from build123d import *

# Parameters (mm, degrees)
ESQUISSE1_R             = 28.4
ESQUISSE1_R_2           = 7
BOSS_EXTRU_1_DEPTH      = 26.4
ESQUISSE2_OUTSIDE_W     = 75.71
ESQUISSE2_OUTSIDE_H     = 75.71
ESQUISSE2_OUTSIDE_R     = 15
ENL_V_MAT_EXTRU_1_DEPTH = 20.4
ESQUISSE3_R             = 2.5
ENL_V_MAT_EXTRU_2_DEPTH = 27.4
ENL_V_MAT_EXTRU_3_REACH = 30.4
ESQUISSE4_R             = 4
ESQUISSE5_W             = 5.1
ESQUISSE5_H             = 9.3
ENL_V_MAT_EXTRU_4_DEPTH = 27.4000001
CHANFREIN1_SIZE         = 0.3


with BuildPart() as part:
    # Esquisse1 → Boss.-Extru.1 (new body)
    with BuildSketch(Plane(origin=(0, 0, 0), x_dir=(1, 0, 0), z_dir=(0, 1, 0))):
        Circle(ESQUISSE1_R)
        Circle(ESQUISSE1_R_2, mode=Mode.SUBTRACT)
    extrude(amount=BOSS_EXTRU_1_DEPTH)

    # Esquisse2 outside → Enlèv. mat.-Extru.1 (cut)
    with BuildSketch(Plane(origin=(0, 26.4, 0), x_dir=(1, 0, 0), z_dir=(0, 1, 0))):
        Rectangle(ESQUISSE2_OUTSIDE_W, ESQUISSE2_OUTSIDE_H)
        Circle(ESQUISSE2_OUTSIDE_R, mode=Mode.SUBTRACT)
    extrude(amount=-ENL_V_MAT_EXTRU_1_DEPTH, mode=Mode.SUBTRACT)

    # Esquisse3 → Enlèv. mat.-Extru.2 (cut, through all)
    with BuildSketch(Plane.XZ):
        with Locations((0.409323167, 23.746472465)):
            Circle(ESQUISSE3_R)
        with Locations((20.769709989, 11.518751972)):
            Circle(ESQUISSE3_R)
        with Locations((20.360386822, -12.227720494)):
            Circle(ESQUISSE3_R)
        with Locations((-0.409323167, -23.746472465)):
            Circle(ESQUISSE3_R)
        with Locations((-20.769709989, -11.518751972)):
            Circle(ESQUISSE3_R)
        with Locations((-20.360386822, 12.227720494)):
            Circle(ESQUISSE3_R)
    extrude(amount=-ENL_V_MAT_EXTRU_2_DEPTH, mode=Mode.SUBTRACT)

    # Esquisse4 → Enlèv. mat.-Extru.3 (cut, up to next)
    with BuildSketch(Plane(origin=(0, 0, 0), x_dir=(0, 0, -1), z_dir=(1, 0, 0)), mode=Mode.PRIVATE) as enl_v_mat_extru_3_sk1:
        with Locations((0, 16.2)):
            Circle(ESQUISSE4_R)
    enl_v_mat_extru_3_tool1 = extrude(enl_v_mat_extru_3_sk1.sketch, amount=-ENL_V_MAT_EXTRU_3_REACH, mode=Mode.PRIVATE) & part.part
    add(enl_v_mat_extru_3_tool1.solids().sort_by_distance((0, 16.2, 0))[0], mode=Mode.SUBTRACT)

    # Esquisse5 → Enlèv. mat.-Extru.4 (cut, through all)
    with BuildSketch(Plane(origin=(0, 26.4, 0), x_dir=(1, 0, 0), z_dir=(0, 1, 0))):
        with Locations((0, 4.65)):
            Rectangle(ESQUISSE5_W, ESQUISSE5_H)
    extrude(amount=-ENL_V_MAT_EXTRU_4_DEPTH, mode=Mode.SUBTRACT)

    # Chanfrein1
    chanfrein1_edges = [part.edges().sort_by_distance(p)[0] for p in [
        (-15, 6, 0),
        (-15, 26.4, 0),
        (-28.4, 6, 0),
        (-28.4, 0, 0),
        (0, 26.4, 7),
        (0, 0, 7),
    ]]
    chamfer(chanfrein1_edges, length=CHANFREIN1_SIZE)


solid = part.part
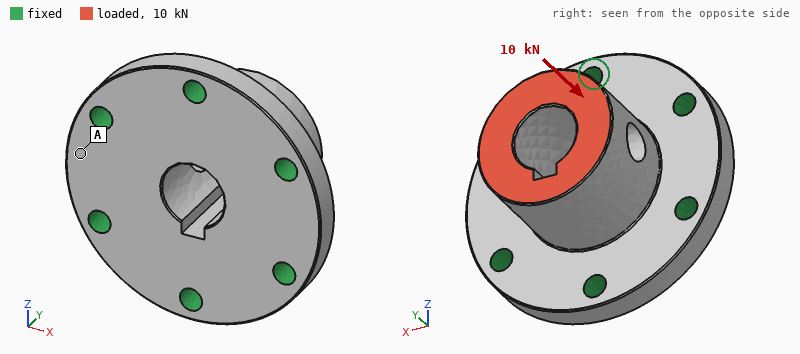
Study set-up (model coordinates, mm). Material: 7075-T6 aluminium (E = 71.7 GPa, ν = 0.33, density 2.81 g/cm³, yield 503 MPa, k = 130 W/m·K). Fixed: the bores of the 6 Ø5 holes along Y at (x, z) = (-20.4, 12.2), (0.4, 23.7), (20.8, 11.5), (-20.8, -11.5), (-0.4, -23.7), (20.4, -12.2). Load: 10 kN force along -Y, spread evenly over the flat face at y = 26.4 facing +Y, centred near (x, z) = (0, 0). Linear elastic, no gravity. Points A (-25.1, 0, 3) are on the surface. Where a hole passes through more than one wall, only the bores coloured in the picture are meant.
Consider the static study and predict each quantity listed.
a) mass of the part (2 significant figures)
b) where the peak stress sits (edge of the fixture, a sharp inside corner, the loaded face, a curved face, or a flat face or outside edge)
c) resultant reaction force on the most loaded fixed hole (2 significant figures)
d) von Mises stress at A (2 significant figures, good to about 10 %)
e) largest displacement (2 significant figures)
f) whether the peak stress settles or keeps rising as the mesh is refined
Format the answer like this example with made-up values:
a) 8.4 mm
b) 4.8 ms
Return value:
a) 68 g
b) edge of the fixture
c) 1.9 kN
d) 15 MPa
e) 26 µm
f) keeps rising
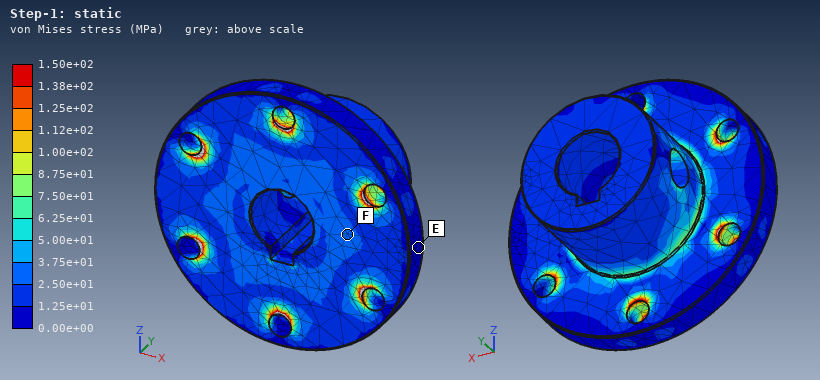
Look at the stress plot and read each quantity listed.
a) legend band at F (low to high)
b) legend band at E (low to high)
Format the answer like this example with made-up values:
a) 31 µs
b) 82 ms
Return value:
a) 2.50e+01 to 3.75e+01 MPa
b) 0.00e+00 to 1.25e+01 MPa
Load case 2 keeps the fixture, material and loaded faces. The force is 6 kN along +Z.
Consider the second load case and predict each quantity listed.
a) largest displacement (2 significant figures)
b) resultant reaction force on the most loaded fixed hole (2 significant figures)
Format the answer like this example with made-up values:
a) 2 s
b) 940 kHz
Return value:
a) 60 µm
b) 2.8 kN
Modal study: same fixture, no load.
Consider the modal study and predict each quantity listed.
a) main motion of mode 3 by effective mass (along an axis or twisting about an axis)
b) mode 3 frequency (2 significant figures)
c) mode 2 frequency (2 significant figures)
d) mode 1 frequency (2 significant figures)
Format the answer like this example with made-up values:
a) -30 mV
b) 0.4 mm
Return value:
a) along Y
b) 18 kHz
c) 15 kHz
d) 15 kHz
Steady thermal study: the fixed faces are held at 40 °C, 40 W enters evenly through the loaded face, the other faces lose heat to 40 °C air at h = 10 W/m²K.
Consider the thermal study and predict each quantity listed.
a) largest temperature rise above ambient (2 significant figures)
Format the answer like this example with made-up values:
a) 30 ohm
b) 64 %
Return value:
a) 20 K
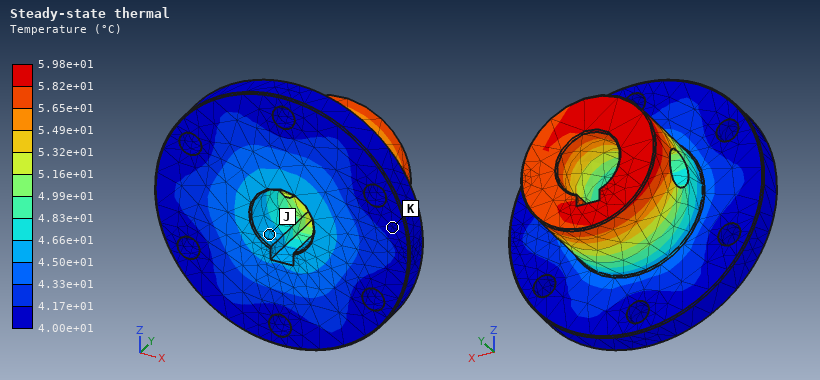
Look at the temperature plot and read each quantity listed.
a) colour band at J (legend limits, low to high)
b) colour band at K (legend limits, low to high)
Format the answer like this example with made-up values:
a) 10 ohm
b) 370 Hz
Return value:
a) 4.50e+01 to 4.66e+01 °C
b) 4.00e+01 to 4.17e+01 °C
